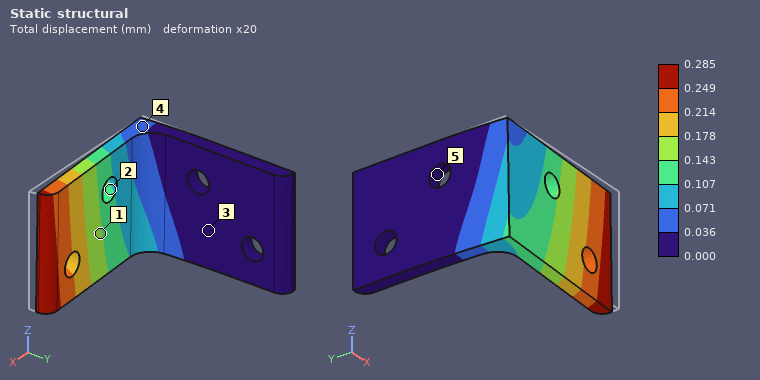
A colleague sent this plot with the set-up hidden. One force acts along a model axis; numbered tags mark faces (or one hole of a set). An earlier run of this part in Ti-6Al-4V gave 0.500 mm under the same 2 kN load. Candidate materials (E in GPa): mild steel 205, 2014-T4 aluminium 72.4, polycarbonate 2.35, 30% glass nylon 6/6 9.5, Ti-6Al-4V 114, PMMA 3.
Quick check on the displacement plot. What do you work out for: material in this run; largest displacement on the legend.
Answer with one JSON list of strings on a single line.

["mild steel", "0.285 mm"]
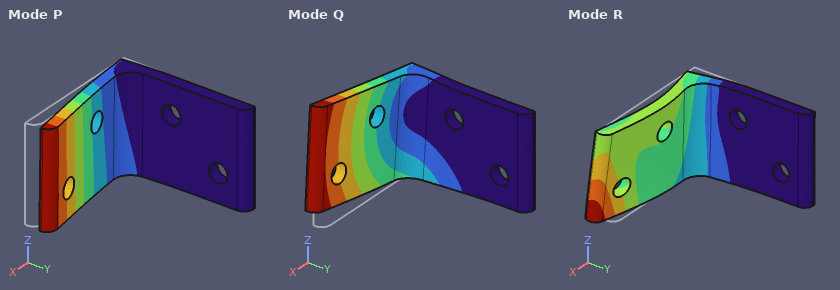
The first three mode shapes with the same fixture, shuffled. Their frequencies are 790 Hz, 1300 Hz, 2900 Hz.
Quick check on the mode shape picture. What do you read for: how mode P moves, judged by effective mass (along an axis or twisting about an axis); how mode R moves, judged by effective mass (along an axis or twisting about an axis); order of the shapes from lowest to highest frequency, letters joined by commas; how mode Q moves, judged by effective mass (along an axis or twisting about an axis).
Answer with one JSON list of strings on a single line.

["along Y", "along X", "P, Q, R", "along Z"]
